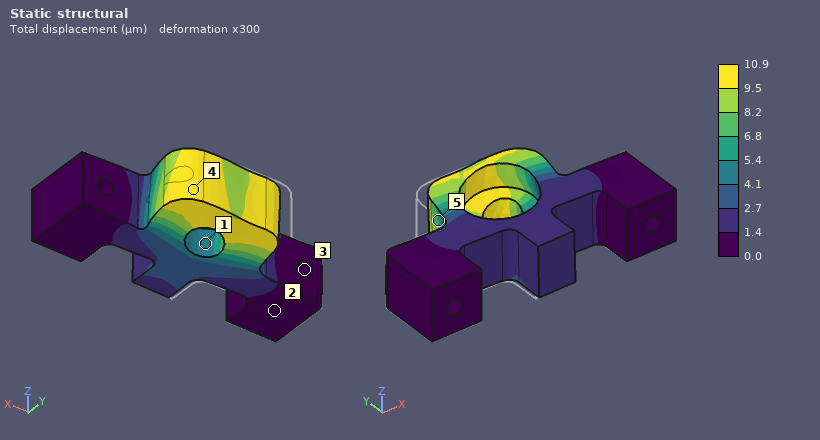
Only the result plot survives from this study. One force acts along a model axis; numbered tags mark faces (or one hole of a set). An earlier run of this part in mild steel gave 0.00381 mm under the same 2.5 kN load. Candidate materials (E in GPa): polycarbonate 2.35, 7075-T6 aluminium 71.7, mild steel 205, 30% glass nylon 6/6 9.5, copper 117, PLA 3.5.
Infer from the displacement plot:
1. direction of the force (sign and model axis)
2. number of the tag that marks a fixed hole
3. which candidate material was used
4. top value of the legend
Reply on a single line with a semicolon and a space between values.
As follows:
+X; 3; 7075-T6 aluminium; 10.9 µm
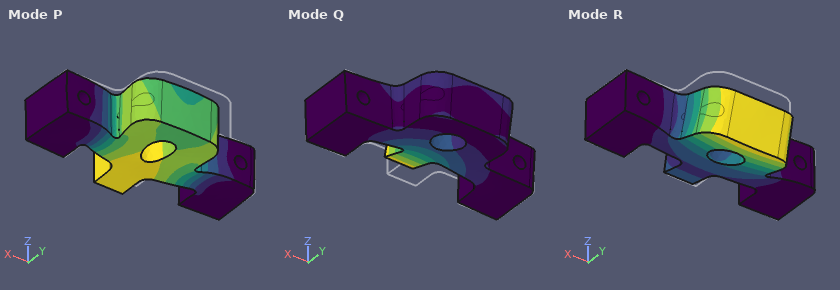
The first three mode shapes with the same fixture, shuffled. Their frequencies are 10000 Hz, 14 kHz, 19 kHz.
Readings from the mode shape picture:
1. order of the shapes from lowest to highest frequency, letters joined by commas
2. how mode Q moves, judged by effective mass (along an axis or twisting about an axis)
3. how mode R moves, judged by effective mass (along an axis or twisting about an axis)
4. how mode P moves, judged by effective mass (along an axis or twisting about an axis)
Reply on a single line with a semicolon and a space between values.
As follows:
R, Q, P; along Z; along Z; along Y
